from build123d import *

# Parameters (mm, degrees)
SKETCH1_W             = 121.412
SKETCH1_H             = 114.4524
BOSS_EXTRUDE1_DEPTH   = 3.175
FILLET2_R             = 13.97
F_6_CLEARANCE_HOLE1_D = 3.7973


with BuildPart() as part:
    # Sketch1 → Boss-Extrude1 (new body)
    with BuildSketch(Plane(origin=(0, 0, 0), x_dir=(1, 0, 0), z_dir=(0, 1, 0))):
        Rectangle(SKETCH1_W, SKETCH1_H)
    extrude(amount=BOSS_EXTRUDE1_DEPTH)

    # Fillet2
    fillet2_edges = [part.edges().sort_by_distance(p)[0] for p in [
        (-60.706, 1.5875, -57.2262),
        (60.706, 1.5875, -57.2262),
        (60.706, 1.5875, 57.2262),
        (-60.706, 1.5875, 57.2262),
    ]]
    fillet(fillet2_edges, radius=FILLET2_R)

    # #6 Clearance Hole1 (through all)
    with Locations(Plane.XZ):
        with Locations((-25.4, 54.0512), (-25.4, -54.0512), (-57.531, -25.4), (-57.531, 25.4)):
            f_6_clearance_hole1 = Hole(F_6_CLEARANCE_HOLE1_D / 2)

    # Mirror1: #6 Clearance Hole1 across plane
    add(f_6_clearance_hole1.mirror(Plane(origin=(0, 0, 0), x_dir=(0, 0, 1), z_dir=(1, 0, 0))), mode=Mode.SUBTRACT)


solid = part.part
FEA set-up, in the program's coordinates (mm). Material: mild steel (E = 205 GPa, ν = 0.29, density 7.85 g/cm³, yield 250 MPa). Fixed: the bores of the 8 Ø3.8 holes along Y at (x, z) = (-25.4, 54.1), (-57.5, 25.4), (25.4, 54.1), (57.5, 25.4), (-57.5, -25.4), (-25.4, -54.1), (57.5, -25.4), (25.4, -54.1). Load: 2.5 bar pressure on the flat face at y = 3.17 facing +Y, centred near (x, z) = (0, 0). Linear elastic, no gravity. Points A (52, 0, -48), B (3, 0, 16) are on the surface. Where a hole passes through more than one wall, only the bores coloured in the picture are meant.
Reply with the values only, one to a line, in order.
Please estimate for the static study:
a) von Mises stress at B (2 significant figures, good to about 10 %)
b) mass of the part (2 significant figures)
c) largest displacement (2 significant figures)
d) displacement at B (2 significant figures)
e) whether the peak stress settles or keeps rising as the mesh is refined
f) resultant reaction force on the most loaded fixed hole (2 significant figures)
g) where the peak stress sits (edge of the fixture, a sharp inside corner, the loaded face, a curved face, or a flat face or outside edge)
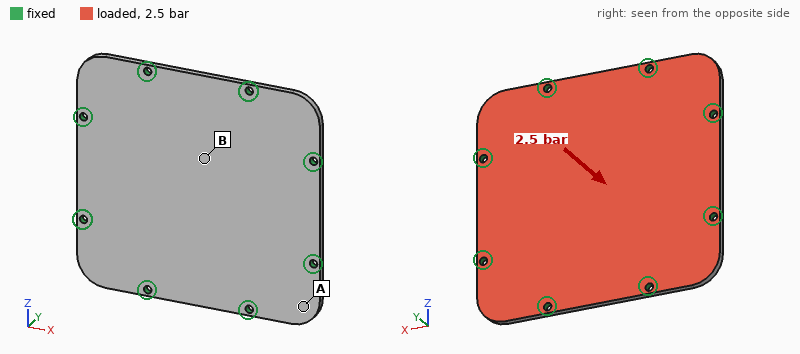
47 MPa
340 g
0.13 mm
0.11 mm
keeps rising
440 N
edge of the fixture
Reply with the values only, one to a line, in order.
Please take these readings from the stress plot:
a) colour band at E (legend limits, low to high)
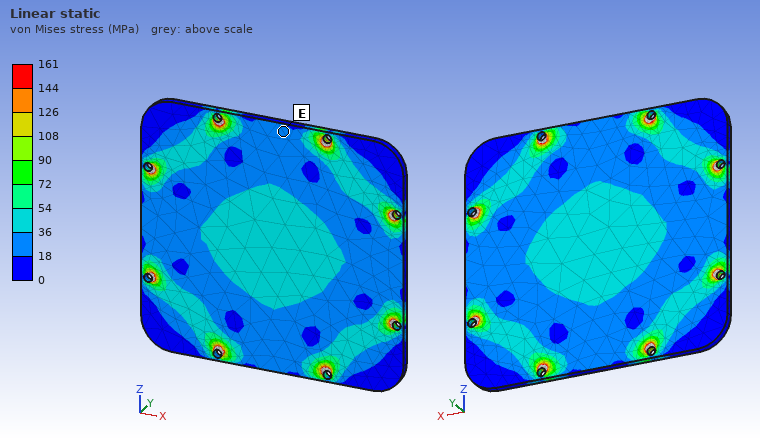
18 to 36 MPa
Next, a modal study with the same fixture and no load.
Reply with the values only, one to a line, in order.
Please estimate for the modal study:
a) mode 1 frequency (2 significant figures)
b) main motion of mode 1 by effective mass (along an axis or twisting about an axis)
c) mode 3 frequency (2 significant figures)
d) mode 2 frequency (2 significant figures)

1700 Hz
along Y
3800 Hz
3600 Hz
